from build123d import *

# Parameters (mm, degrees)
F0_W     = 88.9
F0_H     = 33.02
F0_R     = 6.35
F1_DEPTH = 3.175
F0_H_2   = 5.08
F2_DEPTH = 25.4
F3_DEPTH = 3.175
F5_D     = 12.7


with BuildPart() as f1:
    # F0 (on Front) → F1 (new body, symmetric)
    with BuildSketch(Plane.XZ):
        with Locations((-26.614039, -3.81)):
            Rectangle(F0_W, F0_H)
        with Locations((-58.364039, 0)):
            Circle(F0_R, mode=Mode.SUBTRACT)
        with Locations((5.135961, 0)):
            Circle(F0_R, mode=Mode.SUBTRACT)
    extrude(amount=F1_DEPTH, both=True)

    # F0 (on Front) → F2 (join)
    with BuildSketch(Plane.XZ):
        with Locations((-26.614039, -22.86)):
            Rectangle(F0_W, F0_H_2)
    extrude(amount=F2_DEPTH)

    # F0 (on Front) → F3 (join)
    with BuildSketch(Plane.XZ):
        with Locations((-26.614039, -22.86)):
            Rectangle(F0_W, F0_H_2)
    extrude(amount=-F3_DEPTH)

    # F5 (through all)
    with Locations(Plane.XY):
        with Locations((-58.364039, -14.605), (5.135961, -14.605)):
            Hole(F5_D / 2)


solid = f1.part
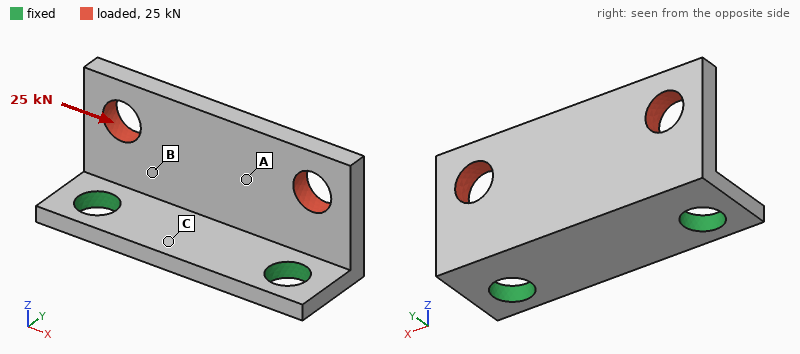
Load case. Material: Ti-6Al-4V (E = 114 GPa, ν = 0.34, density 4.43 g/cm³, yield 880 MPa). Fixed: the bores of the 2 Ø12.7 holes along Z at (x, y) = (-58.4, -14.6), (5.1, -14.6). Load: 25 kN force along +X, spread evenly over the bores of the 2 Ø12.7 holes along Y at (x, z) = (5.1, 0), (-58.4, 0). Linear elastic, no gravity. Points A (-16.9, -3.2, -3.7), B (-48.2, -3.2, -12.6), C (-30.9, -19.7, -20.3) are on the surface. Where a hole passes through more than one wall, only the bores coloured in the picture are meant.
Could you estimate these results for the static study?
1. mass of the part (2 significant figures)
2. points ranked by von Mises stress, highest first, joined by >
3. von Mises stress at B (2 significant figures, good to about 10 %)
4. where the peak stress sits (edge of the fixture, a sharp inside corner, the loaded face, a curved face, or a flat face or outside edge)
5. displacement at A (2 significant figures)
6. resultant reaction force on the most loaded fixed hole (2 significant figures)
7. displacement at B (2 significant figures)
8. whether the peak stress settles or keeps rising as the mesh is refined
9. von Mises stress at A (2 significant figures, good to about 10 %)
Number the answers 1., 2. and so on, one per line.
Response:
1. 130 g
2. B > A > C
3. 190 MPa
4. edge of the fixture
5. 0.093 mm
6. 16 kN
7. 0.076 mm
8. keeps rising
9. 130 MPa
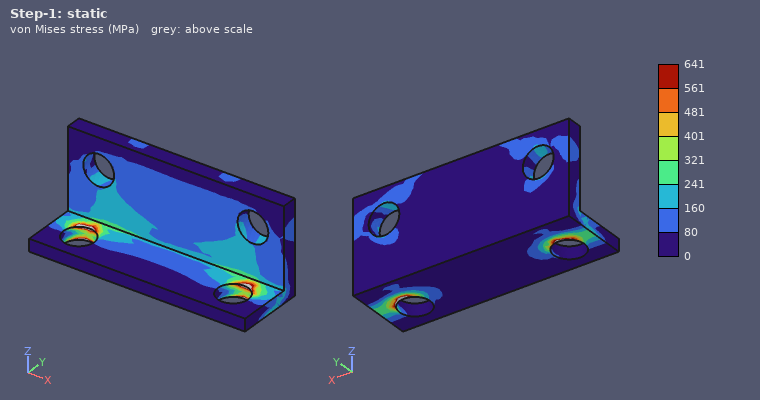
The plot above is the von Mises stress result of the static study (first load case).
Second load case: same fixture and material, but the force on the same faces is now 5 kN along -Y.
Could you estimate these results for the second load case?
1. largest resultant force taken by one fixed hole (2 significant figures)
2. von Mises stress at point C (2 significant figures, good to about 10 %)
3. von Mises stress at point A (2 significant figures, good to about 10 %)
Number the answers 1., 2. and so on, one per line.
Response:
1. 2.5 kN
2. 64 MPa
3. 57 MPa
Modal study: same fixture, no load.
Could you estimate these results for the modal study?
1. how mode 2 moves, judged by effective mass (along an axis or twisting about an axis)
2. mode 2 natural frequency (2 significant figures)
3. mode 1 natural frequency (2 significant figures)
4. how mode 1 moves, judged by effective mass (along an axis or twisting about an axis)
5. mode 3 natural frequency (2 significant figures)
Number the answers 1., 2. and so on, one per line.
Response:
1. twisting about Z
2. 4100 Hz
3. 2300 Hz
4. along Y
5. 7600 Hz
